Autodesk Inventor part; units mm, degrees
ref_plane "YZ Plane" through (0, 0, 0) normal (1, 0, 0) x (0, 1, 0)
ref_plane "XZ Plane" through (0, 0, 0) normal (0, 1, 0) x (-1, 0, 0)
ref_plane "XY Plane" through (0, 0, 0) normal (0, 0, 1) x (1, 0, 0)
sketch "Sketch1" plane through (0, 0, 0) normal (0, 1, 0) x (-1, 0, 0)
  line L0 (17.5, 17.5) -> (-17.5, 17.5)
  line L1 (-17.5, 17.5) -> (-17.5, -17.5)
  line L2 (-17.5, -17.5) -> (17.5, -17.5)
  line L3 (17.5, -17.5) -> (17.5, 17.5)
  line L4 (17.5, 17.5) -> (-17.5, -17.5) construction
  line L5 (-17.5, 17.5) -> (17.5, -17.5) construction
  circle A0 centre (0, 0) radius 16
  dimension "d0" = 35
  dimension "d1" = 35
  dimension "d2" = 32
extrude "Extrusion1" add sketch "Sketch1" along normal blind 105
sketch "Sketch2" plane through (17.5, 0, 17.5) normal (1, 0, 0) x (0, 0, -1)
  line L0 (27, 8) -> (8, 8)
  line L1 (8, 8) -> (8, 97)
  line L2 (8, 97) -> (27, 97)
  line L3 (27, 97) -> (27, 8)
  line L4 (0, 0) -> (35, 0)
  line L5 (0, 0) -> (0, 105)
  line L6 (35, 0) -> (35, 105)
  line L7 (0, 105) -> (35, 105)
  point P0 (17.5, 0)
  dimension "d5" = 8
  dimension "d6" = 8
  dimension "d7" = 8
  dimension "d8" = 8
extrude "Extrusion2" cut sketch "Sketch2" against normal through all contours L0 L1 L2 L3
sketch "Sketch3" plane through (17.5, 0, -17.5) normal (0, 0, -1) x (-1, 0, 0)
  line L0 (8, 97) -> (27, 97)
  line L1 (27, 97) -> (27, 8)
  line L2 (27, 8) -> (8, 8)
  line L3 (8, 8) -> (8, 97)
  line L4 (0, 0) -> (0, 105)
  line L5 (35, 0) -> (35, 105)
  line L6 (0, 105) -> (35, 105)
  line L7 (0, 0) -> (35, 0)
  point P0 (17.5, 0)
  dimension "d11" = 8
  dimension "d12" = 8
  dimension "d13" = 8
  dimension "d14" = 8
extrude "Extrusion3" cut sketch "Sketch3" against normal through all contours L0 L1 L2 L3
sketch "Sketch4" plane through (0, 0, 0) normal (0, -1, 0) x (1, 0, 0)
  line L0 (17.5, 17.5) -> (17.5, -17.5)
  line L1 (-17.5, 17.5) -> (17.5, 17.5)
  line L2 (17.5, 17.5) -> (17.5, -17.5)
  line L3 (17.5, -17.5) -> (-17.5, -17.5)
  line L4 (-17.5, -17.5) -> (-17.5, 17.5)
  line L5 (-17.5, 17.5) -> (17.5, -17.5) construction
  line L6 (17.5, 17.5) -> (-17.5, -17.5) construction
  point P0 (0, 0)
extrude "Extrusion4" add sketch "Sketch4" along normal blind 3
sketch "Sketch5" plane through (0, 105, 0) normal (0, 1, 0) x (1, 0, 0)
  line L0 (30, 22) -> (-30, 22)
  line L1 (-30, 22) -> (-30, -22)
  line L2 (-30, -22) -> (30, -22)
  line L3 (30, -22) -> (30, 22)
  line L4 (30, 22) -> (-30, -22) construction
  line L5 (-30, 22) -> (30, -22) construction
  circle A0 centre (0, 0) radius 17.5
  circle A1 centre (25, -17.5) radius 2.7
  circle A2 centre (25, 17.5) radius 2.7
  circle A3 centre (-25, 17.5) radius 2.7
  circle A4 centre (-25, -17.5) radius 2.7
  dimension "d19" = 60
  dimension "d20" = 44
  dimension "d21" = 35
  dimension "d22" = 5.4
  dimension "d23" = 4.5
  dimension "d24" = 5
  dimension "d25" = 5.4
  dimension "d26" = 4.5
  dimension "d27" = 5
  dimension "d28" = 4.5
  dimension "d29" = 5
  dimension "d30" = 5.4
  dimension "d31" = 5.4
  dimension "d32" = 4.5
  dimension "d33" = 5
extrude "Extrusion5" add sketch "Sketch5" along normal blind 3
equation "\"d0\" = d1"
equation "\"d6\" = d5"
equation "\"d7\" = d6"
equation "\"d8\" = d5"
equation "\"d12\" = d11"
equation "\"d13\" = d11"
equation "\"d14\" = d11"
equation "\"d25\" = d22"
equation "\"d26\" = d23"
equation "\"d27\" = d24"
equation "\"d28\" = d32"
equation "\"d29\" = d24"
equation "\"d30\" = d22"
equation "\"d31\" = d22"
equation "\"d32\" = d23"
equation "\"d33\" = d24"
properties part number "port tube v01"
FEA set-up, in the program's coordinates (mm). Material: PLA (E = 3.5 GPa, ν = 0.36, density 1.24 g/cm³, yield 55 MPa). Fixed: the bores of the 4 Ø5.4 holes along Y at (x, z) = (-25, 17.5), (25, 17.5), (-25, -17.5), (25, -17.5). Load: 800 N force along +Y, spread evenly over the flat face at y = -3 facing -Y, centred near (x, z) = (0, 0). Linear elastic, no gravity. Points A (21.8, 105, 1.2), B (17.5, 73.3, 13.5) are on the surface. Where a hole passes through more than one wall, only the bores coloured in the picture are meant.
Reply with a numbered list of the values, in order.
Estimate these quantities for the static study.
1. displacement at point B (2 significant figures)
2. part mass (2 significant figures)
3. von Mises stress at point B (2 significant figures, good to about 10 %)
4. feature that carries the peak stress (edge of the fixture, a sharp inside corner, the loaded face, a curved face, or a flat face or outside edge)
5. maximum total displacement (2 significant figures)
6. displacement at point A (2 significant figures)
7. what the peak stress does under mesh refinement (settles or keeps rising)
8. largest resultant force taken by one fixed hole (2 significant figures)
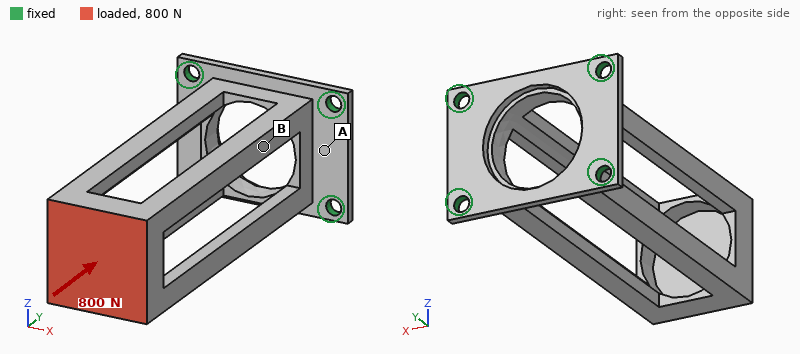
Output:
1. 0.20 mm
2. 44 g
3. 5.2 MPa
4. edge of the fixture
5. 0.42 mm
6. 0.088 mm
7. keeps rising
8. 230 N
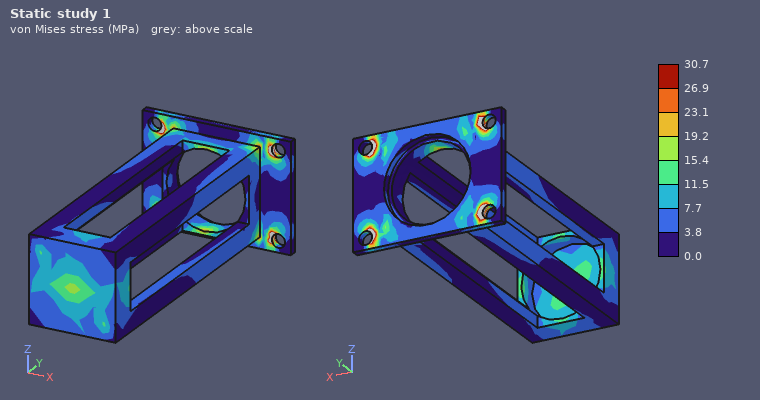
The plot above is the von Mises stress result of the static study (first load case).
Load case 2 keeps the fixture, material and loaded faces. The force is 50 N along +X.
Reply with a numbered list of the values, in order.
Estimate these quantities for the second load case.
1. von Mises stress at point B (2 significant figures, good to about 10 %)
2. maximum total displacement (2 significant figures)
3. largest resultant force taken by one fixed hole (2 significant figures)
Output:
1. 4.6 MPa
2. 1.4 mm
3. 70 N
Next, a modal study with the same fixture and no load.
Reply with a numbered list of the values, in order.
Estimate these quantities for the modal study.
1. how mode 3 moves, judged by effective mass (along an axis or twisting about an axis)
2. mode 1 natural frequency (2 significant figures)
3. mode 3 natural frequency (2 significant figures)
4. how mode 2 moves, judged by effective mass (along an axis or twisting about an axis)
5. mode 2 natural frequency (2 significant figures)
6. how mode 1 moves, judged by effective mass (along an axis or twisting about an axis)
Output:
1. twisting about Y
2. 220 Hz
3. 440 Hz
4. along X
5. 230 Hz
6. along Z
